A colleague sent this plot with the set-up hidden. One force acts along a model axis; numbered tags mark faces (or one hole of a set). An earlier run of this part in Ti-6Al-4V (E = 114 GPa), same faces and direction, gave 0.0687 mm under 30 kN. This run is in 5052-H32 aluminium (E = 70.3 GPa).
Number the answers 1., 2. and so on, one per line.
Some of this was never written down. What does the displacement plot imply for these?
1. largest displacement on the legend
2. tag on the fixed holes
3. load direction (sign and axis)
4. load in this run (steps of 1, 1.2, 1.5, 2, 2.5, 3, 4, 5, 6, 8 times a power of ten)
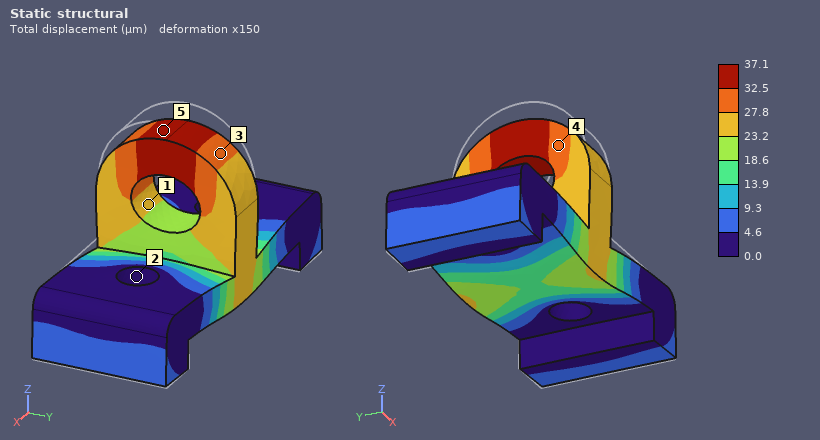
1. 37.1 µm
2. 2
3. -Z
4. 10 kN
